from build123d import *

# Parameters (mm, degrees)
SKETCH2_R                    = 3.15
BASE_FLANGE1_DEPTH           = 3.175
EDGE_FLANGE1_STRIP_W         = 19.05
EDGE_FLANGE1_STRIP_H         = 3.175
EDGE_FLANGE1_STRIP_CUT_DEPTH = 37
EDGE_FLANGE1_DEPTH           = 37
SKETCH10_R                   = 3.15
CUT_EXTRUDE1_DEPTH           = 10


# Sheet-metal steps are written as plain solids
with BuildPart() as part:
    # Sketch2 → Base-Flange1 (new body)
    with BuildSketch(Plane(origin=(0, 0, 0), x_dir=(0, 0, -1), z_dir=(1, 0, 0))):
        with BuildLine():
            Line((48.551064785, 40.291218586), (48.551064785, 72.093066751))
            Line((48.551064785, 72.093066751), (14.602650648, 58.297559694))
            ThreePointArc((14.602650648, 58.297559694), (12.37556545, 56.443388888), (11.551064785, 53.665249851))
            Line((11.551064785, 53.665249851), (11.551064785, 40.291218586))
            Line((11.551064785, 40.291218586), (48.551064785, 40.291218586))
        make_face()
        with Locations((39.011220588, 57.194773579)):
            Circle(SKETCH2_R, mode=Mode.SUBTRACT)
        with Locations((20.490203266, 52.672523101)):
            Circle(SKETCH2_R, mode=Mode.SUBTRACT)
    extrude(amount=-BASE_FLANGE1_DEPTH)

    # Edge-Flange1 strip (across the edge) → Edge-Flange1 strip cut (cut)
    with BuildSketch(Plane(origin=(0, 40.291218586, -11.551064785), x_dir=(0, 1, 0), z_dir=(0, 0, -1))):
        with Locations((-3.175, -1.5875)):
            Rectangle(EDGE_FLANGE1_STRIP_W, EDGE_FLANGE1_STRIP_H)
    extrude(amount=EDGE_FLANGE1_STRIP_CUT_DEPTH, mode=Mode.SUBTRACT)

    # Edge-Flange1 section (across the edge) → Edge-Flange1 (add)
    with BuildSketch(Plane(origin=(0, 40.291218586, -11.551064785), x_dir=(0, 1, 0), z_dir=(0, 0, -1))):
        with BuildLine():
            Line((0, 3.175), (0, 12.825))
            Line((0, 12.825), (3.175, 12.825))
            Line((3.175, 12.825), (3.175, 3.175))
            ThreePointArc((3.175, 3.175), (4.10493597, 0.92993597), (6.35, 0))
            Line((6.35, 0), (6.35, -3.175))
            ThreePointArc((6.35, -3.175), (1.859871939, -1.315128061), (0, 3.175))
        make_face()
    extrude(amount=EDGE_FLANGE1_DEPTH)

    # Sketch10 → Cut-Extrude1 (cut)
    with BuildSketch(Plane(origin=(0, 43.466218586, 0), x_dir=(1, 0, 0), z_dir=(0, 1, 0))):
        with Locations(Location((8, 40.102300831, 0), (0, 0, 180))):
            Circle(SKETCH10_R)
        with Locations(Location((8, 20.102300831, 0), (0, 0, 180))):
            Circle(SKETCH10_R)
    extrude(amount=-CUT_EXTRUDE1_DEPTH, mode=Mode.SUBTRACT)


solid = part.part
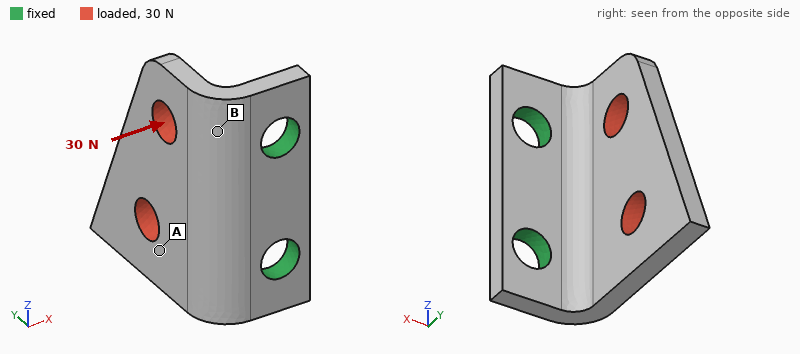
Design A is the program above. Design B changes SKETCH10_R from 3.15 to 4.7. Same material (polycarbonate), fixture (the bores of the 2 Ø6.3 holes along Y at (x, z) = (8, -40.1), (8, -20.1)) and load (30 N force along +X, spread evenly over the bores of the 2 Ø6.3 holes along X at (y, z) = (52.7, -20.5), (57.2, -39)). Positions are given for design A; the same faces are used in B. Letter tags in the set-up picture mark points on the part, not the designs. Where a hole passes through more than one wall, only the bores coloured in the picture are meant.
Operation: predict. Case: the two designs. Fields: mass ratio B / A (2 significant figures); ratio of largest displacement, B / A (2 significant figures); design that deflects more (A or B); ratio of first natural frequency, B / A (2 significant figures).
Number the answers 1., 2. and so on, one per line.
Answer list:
1. 0.93
2. 0.85
3. A
4. 1.1
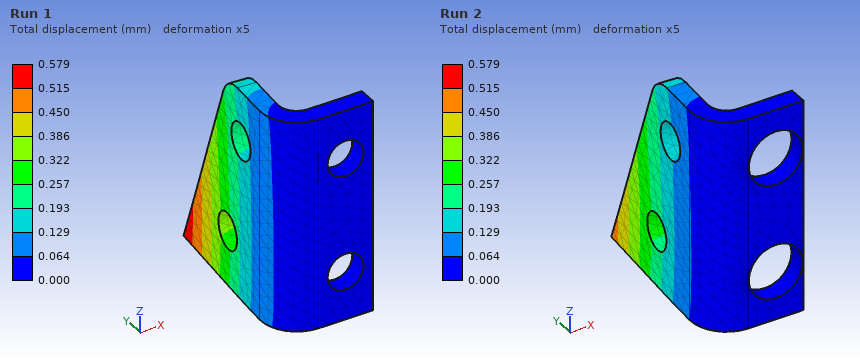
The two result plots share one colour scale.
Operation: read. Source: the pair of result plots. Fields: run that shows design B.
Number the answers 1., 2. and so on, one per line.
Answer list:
1. Run 2
